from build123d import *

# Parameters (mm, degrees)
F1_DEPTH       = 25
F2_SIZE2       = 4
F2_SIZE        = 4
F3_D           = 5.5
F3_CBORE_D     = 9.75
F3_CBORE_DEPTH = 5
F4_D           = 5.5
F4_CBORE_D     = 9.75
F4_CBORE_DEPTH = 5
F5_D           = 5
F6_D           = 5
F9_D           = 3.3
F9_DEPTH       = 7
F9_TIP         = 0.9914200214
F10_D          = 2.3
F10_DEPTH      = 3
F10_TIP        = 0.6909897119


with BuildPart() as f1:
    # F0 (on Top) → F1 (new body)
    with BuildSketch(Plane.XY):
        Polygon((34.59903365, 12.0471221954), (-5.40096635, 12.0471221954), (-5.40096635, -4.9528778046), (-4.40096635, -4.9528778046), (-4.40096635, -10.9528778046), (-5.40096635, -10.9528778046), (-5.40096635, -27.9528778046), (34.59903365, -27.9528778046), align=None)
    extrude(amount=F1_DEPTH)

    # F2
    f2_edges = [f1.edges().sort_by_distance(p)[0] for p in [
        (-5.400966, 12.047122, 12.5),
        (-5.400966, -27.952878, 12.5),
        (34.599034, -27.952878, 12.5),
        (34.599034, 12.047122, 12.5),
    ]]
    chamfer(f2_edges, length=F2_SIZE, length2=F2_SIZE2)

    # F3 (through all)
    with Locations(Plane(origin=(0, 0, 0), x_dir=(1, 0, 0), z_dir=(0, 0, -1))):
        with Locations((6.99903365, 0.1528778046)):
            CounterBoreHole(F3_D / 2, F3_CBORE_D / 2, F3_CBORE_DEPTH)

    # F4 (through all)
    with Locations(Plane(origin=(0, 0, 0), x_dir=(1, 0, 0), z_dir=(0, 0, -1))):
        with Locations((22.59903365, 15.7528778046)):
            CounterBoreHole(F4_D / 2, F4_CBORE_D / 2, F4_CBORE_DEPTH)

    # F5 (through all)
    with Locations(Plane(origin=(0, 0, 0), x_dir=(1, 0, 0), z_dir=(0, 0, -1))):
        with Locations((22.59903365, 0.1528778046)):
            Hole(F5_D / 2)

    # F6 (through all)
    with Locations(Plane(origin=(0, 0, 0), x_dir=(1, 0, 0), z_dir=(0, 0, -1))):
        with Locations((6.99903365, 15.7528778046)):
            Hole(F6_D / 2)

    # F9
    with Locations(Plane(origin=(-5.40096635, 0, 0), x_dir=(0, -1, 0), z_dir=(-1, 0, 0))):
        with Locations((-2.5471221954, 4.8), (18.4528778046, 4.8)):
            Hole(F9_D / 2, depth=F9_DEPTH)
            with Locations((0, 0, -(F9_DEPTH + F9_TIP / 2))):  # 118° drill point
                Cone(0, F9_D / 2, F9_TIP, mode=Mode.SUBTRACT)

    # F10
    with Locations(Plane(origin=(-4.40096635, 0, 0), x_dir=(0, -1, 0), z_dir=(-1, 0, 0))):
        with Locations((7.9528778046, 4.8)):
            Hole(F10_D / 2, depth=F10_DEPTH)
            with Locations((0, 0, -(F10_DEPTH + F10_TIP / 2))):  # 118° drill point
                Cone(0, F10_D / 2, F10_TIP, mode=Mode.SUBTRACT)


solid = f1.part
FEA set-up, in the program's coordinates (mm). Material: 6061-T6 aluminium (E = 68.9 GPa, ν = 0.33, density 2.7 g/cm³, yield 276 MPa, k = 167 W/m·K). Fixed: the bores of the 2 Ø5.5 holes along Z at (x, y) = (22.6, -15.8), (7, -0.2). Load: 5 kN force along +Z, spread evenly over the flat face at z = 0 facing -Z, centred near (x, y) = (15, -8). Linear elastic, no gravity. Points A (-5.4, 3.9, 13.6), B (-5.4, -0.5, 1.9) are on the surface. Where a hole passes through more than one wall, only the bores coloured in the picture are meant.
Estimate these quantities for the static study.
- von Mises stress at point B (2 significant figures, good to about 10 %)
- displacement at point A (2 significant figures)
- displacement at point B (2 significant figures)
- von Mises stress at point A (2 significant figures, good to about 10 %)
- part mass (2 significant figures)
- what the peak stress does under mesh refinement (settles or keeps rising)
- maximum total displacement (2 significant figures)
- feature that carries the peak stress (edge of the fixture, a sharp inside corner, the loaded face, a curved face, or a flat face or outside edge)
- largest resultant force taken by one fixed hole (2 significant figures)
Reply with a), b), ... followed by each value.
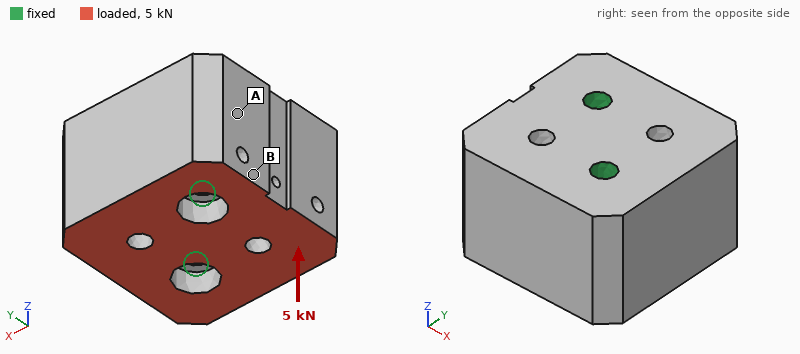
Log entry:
a) 6.1 MPa
b) 0.93 µm
c) 1.7 µm
d) 1.7 MPa
e) 98 g
f) keeps rising
g) 4.3 µm
h) edge of the fixture
i) 2.5 kN
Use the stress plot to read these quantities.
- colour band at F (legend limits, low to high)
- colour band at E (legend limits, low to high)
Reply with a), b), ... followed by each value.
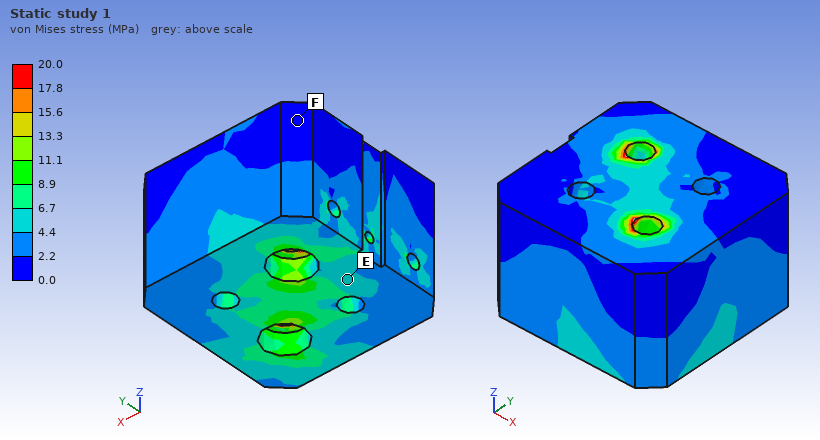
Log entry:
a) 0.0 to 2.2 MPa
b) 4.4 to 6.7 MPa
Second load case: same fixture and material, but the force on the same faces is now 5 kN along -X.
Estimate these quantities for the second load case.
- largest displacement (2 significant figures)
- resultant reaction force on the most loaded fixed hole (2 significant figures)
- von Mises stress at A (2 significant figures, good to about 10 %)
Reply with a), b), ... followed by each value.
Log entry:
a) 8.4 µm
b) 2.8 kN
c) 6.0 MPa
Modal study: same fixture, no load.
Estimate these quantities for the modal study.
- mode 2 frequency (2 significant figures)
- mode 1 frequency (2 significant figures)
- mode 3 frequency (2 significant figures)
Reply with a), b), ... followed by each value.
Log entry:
a) 26 kHz
b) 20 kHz
c) 26 kHz
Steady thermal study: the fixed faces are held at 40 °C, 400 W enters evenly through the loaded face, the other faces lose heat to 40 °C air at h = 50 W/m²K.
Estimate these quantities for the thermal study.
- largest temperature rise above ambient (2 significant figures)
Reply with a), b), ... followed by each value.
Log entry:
a) 38 K
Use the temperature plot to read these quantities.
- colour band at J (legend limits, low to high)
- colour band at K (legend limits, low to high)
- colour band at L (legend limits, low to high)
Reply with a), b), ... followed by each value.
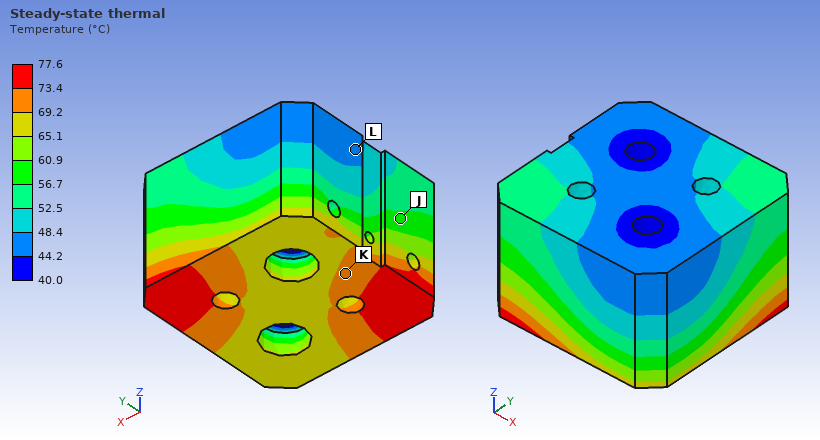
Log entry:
a) 56.7 to 60.9 °C
b) 69.2 to 73.4 °C
c) 44.2 to 48.4 °C
